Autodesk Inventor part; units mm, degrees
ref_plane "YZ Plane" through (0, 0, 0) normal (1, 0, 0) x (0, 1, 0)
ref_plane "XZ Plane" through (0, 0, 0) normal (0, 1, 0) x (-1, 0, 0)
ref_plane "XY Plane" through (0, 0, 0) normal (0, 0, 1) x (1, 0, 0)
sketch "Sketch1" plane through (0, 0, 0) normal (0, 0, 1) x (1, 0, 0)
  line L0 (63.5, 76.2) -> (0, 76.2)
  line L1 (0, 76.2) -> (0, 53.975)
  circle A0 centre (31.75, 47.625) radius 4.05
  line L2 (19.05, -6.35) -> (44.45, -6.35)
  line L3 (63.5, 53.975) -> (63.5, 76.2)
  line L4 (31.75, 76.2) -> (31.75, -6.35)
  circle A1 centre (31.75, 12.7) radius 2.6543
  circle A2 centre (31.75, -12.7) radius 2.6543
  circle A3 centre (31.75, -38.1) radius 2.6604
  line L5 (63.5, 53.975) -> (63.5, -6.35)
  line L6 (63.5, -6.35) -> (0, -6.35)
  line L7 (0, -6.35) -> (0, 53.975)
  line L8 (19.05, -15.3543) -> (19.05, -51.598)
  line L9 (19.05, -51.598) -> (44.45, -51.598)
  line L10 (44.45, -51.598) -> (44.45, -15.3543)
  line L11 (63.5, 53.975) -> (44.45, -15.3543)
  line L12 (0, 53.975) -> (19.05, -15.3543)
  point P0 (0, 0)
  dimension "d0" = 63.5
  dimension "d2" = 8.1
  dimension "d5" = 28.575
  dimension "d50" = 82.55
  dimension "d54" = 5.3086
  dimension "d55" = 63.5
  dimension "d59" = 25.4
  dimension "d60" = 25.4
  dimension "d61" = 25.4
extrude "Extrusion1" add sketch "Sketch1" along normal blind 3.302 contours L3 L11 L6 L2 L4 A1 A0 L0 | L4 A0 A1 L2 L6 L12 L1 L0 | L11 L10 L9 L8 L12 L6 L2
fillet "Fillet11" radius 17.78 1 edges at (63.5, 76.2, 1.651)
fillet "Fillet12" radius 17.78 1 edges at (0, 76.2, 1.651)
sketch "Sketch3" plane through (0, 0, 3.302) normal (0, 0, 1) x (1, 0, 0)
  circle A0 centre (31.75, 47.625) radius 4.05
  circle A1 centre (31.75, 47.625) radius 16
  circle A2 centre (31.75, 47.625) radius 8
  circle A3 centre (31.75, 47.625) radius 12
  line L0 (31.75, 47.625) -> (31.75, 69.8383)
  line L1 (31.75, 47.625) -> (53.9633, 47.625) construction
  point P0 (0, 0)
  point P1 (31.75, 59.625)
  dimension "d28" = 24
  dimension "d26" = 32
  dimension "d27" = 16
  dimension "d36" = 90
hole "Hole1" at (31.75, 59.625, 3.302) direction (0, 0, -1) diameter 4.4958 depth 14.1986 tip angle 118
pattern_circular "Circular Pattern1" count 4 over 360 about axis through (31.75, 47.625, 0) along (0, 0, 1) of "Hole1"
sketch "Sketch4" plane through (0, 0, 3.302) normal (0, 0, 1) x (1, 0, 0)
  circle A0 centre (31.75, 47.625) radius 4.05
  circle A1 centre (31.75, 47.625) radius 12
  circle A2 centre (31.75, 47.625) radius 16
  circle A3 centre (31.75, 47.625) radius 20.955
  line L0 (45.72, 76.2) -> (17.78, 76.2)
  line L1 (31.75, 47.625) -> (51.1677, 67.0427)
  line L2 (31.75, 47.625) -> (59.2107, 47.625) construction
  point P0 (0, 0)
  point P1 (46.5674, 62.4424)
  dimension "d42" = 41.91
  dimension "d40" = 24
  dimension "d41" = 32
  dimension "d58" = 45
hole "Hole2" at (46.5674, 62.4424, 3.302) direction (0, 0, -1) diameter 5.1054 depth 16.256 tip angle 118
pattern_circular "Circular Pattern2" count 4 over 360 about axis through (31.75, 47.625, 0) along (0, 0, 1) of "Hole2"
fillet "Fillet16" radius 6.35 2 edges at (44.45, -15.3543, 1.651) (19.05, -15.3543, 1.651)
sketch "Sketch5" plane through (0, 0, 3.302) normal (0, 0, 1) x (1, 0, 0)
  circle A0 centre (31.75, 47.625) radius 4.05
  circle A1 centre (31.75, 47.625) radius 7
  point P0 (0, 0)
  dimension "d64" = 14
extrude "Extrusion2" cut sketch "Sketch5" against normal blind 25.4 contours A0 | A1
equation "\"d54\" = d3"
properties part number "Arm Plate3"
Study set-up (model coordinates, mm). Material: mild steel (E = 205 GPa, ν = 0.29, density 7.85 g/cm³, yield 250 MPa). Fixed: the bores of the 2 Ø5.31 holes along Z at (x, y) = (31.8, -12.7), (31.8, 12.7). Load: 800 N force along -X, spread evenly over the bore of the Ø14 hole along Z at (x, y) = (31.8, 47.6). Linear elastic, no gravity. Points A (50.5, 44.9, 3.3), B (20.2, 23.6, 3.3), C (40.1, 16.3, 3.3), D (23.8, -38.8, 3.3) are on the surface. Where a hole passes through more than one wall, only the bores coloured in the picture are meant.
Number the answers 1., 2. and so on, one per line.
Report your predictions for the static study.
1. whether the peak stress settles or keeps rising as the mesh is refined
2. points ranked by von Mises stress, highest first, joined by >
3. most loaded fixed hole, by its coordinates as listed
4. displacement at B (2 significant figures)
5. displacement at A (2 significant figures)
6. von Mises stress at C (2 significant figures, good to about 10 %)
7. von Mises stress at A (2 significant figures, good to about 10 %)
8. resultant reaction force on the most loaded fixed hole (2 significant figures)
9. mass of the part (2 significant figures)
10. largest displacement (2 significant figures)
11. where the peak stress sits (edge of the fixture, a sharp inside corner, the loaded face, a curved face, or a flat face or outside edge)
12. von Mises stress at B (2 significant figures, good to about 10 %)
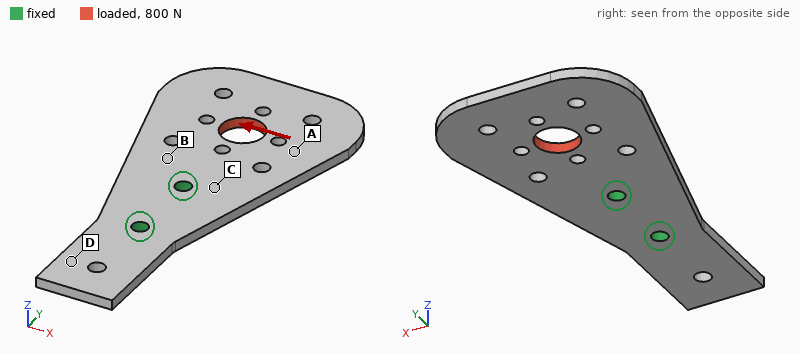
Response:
1. keeps rising
2. C > B > A > D
3. (31.8, 12.7)
4. 4.8 µm
5. 14 µm
6. 20 MPa
7. 7.9 MPa
8. 1.7 kN
9. 130 g
10. 24 µm
11. edge of the fixture
12. 16 MPa
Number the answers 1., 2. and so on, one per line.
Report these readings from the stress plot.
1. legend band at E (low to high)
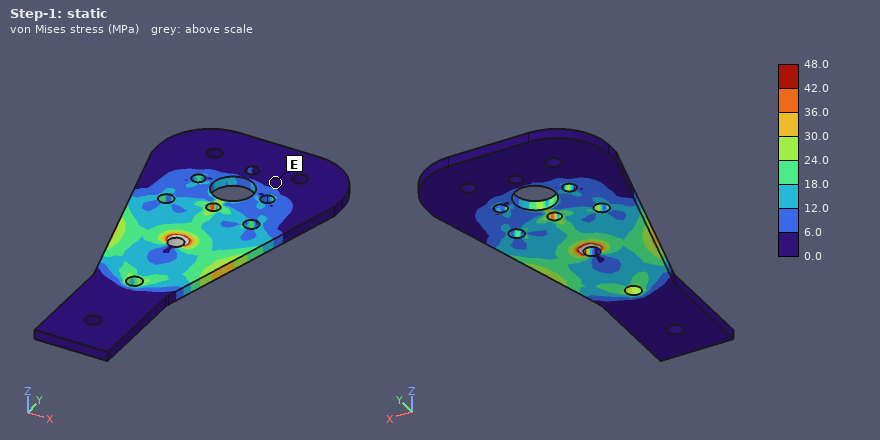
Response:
1. 0.0 to 6.0 MPa
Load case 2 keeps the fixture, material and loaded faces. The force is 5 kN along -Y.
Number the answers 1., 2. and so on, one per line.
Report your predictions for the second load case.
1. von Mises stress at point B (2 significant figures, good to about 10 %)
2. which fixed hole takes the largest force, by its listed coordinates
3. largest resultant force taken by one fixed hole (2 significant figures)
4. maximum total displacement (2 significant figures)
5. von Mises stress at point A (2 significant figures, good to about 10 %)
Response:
1. 31 MPa
2. (31.8, 12.7)
3. 3.7 kN
4. 14 µm
5. 18 MPa
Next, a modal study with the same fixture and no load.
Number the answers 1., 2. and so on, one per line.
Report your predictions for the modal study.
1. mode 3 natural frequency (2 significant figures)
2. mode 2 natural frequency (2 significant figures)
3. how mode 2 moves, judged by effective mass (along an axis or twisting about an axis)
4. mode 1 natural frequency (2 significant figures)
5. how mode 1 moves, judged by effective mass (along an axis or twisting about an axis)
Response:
1. 1900 Hz
2. 1200 Hz
3. twisting about Y
4. 600 Hz
5. along Z
